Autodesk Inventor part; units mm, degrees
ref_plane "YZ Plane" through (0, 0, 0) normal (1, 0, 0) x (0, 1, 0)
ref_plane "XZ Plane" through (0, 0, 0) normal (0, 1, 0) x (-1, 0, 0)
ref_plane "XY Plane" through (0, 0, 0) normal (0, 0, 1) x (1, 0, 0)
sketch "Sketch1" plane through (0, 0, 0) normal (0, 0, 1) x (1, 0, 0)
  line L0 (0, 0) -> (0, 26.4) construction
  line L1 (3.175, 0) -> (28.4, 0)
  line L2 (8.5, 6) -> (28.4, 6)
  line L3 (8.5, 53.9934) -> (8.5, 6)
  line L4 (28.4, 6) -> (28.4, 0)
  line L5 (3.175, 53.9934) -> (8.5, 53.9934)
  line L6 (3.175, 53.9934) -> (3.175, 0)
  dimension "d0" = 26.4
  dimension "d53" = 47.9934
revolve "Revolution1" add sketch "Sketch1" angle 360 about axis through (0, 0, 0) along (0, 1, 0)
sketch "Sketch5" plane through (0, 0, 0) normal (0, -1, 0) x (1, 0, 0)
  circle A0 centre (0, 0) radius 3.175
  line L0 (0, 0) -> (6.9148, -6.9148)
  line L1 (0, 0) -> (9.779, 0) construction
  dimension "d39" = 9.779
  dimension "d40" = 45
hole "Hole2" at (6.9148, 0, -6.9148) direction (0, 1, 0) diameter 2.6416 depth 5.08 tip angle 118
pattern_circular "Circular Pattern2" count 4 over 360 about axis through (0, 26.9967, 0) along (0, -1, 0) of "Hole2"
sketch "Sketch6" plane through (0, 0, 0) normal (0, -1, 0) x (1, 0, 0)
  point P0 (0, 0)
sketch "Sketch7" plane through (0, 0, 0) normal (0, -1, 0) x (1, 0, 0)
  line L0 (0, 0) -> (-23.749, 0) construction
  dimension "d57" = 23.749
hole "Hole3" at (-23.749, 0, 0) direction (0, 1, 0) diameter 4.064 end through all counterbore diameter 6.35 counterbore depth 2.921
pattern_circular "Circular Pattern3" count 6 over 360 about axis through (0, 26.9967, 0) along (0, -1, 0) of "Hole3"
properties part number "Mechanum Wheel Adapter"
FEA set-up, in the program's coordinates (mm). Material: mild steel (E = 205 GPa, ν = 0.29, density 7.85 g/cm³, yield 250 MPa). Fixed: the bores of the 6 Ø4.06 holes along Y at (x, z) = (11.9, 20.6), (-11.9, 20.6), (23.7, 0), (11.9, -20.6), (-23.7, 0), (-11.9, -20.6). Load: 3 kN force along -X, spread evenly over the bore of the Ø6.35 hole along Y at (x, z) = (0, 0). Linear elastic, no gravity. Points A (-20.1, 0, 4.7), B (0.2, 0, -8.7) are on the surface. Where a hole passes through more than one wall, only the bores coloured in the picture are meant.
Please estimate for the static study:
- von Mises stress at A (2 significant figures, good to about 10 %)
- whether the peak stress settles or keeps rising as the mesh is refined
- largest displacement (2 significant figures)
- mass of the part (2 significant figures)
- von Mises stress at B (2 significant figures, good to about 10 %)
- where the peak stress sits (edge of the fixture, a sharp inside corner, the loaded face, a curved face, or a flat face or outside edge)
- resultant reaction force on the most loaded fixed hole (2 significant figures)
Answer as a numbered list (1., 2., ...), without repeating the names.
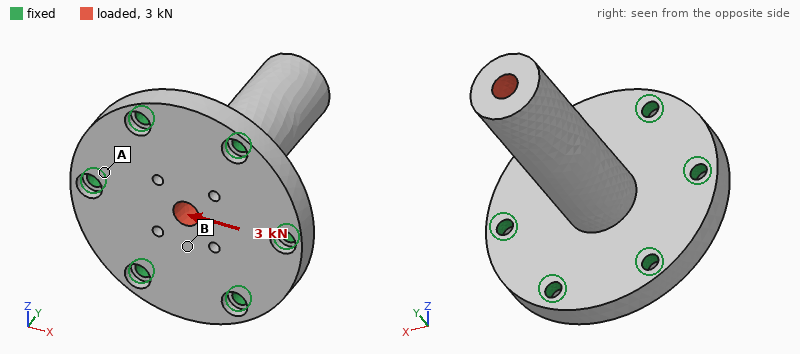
1. 35 MPa
2. keeps rising
3. 0.12 mm
4. 180 g
5. 69 MPa
6. edge of the fixture
7. 1.2 kN
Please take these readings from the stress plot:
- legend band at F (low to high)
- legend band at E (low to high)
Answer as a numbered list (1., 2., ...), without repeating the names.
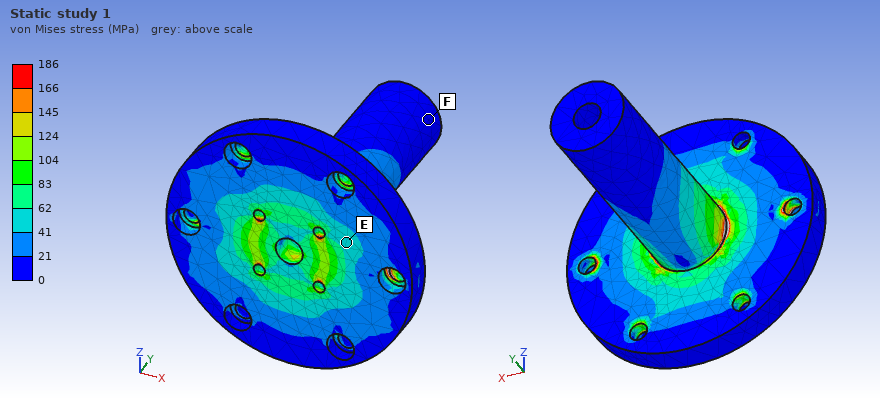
1. 0 to 21 MPa
2. 41 to 62 MPa
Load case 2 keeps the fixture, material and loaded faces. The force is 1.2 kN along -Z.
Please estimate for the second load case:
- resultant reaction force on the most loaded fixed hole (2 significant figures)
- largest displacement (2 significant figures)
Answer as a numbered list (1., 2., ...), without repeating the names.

1. 420 N
2. 48 µm
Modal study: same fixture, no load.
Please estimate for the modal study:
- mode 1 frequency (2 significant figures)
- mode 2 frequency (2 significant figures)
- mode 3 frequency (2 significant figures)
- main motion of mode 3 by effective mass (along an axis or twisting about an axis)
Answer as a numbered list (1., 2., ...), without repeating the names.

1. 3400 Hz
2. 3400 Hz
3. 9200 Hz
4. along Y
